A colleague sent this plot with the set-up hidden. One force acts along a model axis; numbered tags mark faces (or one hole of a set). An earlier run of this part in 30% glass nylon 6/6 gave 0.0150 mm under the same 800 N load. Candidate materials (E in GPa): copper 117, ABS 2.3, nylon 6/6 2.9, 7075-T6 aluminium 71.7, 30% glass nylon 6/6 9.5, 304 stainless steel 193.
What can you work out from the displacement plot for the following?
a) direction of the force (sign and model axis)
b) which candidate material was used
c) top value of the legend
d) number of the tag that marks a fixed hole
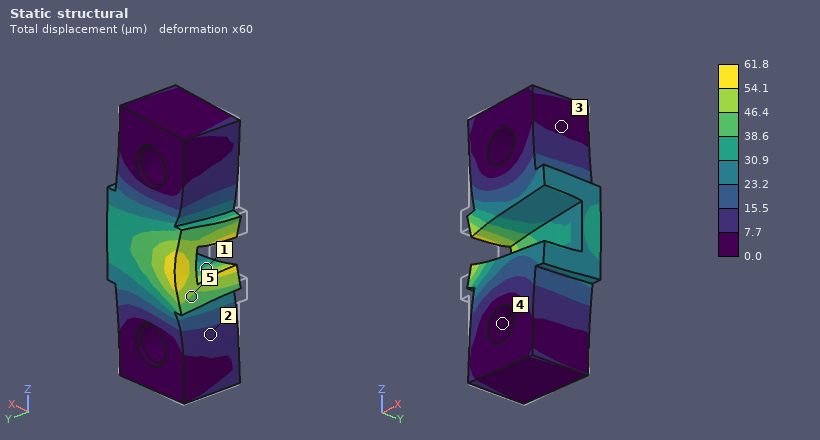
+X
ABS
61.8 µm
4
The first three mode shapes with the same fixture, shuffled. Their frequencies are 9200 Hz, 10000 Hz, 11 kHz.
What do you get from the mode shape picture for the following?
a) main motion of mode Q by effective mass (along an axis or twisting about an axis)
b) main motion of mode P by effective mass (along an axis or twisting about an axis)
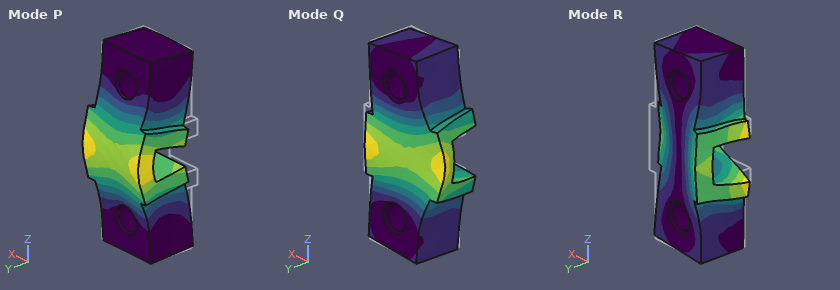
along X
along Y
